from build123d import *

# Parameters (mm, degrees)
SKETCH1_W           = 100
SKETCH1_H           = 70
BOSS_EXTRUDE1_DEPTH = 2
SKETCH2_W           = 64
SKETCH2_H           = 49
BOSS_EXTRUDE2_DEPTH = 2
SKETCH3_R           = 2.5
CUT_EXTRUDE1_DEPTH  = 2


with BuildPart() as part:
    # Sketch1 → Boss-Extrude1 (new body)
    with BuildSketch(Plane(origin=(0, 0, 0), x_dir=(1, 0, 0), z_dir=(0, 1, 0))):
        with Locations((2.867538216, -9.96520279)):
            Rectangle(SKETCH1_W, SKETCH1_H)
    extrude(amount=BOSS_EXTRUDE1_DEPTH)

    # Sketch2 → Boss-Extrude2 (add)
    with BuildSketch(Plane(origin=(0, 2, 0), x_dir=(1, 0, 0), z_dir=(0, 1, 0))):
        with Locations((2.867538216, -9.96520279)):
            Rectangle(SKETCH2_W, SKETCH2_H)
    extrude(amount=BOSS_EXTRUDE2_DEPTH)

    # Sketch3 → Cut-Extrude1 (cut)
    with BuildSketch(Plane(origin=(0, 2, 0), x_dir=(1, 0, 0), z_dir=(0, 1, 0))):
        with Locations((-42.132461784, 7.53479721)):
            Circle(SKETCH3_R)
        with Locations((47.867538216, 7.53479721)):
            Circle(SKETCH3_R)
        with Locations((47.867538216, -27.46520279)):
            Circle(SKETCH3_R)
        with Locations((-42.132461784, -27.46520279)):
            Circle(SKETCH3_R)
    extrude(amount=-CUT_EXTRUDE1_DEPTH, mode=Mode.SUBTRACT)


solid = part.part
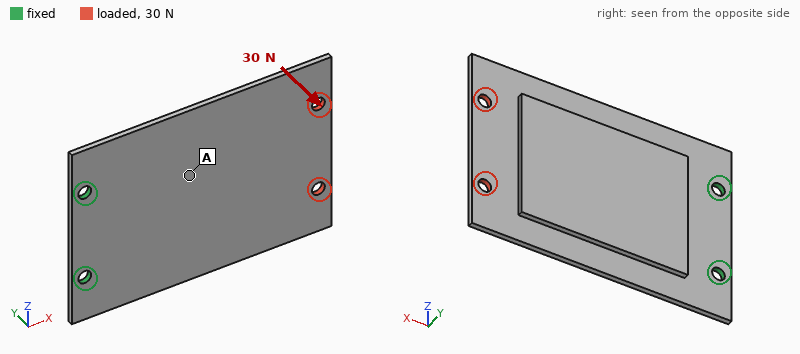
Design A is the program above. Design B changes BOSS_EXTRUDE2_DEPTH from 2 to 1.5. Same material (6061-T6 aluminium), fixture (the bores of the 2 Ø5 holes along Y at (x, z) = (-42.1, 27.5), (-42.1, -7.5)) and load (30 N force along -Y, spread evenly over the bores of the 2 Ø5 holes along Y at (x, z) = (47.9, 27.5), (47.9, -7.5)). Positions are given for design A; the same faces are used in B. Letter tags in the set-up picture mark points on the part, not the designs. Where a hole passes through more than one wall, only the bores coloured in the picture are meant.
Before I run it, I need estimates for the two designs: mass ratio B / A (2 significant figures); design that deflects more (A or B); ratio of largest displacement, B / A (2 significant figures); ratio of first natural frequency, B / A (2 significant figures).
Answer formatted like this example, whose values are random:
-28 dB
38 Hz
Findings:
0.92
B
1.1
1.0
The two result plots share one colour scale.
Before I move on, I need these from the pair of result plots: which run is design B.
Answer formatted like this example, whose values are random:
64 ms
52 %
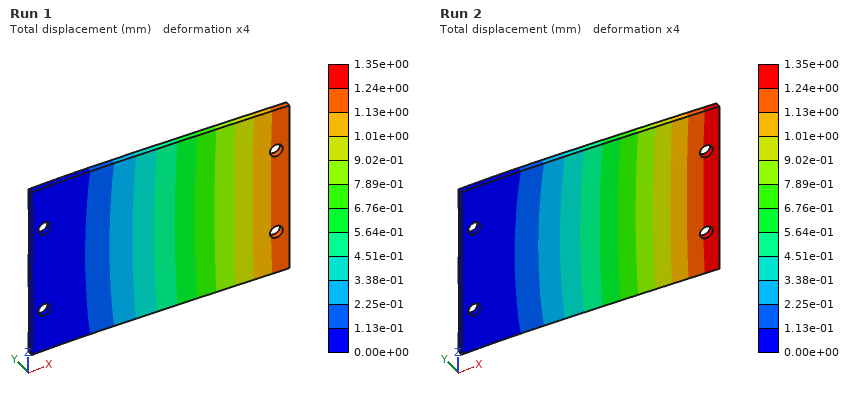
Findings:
Run 2
